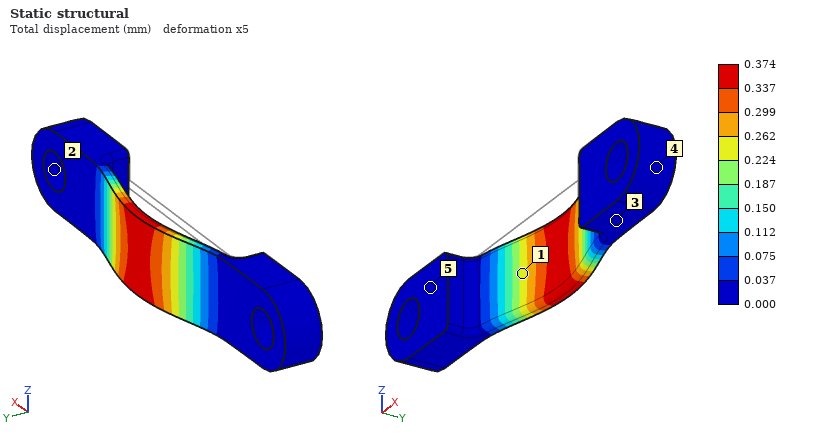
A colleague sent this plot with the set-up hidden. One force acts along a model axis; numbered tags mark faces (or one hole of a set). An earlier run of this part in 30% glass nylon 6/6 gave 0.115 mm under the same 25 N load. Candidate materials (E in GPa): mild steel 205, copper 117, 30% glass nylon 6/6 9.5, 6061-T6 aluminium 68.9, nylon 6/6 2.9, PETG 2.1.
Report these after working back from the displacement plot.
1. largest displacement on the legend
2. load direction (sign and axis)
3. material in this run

0.374 mm
+Y
nylon 6/6
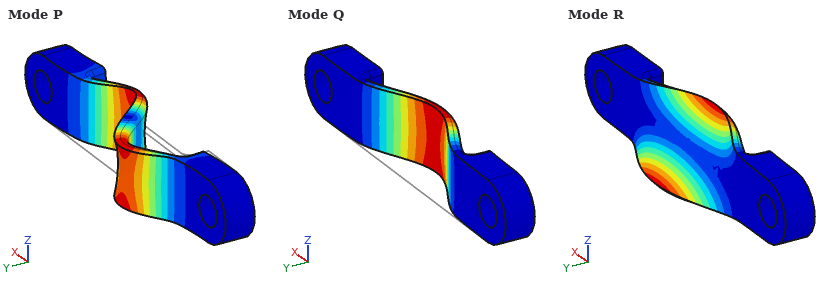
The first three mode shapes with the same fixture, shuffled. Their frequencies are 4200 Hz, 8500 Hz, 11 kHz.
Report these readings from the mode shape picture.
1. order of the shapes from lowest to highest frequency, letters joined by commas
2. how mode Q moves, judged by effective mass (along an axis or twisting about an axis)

Q, R, P
along Y
